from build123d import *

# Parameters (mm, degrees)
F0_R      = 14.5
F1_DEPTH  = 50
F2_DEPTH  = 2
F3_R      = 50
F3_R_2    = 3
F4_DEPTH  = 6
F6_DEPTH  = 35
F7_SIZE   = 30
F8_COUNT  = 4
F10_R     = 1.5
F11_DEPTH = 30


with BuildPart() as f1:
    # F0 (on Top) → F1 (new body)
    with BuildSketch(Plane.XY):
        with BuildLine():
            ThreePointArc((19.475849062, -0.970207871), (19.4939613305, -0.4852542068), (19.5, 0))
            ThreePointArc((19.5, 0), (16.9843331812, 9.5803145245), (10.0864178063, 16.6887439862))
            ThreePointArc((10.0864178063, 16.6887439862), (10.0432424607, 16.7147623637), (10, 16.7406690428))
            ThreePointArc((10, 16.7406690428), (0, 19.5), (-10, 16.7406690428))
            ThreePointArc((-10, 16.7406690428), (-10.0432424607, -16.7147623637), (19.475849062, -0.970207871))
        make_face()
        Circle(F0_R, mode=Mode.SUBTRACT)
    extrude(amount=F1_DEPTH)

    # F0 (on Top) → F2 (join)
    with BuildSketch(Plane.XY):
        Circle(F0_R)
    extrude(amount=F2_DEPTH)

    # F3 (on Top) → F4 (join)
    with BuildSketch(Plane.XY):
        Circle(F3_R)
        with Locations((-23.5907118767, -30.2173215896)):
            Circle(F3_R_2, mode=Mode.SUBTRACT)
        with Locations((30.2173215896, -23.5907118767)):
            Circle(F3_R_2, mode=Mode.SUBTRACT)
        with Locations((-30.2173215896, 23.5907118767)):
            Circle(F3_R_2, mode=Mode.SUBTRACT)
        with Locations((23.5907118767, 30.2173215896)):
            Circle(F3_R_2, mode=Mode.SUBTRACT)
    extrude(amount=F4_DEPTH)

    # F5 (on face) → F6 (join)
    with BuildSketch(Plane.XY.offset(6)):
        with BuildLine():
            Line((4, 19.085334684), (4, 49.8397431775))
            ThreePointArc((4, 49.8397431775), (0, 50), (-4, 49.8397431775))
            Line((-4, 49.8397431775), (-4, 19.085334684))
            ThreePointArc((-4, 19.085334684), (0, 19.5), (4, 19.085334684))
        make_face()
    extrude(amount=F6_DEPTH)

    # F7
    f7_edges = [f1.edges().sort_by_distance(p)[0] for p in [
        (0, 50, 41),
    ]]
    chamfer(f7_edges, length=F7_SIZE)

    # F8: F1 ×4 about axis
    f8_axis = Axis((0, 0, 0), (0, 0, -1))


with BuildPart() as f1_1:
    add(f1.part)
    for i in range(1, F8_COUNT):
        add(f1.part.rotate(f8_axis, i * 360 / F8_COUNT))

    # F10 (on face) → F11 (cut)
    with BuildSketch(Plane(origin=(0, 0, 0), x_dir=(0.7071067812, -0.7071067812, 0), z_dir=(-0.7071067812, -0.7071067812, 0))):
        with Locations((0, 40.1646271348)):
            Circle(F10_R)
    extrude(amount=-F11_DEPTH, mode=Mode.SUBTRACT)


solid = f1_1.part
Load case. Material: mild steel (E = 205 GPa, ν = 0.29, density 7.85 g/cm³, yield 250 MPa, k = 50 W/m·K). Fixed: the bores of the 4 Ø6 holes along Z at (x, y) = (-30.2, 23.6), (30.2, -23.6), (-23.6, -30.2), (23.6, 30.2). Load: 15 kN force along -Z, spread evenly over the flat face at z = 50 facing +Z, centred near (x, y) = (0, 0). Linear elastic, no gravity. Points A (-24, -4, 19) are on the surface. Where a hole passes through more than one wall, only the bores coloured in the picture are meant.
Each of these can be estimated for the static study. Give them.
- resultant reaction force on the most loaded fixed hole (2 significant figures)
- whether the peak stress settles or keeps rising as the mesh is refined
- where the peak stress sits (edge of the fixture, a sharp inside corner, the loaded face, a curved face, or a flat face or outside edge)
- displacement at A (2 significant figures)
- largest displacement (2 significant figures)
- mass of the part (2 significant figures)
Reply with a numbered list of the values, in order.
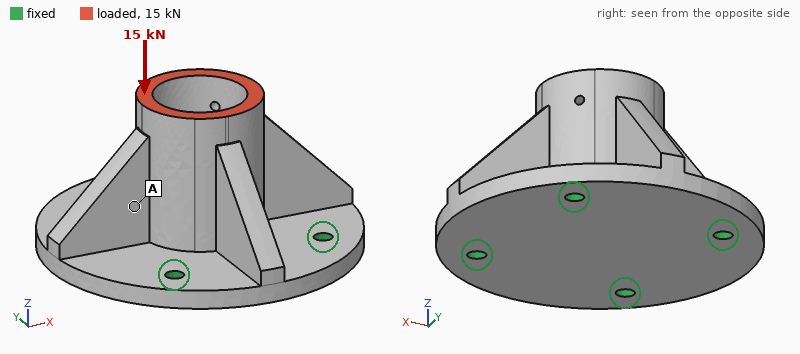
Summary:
1. 3.8 kN
2. keeps rising
3. edge of the fixture
4. 23 µm
5. 27 µm
6. 700 g
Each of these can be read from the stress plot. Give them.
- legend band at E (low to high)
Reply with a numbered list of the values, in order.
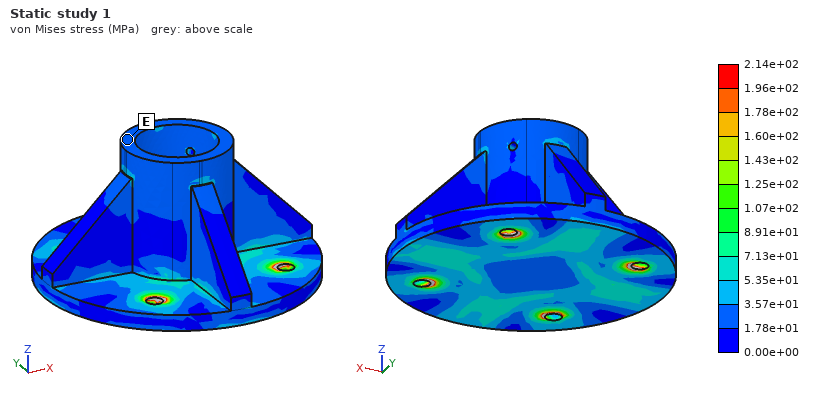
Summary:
1. 1.78e+01 to 3.57e+01 MPa
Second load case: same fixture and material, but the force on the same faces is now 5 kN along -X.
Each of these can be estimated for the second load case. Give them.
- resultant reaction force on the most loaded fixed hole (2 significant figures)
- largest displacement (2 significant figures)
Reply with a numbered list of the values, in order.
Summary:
1. 2.8 kN
2. 42 µm
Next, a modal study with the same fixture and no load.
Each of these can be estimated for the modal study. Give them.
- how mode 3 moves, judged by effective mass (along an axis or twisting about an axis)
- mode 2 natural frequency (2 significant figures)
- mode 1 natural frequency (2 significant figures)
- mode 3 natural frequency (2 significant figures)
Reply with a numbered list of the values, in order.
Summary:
1. along Z
2. 4800 Hz
3. 4800 Hz
4. 5500 Hz
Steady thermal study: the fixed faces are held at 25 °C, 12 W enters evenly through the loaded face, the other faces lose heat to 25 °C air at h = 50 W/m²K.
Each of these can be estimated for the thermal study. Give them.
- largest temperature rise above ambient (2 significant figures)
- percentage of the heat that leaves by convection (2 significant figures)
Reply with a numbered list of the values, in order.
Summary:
1. 14 K
2. 48 %
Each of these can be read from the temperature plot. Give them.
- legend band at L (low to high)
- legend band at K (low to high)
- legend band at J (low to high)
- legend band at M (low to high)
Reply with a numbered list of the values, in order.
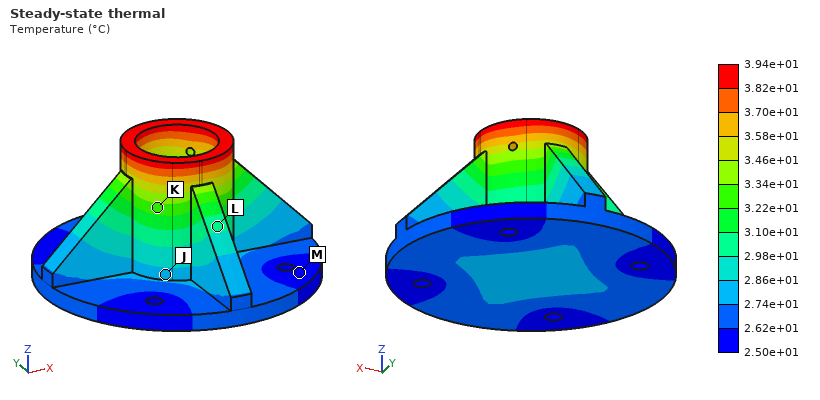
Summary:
1. 2.98e+01 to 3.10e+01 °C
2. 3.22e+01 to 3.34e+01 °C
3. 2.74e+01 to 2.86e+01 °C
4. 2.50e+01 to 2.62e+01 °C
